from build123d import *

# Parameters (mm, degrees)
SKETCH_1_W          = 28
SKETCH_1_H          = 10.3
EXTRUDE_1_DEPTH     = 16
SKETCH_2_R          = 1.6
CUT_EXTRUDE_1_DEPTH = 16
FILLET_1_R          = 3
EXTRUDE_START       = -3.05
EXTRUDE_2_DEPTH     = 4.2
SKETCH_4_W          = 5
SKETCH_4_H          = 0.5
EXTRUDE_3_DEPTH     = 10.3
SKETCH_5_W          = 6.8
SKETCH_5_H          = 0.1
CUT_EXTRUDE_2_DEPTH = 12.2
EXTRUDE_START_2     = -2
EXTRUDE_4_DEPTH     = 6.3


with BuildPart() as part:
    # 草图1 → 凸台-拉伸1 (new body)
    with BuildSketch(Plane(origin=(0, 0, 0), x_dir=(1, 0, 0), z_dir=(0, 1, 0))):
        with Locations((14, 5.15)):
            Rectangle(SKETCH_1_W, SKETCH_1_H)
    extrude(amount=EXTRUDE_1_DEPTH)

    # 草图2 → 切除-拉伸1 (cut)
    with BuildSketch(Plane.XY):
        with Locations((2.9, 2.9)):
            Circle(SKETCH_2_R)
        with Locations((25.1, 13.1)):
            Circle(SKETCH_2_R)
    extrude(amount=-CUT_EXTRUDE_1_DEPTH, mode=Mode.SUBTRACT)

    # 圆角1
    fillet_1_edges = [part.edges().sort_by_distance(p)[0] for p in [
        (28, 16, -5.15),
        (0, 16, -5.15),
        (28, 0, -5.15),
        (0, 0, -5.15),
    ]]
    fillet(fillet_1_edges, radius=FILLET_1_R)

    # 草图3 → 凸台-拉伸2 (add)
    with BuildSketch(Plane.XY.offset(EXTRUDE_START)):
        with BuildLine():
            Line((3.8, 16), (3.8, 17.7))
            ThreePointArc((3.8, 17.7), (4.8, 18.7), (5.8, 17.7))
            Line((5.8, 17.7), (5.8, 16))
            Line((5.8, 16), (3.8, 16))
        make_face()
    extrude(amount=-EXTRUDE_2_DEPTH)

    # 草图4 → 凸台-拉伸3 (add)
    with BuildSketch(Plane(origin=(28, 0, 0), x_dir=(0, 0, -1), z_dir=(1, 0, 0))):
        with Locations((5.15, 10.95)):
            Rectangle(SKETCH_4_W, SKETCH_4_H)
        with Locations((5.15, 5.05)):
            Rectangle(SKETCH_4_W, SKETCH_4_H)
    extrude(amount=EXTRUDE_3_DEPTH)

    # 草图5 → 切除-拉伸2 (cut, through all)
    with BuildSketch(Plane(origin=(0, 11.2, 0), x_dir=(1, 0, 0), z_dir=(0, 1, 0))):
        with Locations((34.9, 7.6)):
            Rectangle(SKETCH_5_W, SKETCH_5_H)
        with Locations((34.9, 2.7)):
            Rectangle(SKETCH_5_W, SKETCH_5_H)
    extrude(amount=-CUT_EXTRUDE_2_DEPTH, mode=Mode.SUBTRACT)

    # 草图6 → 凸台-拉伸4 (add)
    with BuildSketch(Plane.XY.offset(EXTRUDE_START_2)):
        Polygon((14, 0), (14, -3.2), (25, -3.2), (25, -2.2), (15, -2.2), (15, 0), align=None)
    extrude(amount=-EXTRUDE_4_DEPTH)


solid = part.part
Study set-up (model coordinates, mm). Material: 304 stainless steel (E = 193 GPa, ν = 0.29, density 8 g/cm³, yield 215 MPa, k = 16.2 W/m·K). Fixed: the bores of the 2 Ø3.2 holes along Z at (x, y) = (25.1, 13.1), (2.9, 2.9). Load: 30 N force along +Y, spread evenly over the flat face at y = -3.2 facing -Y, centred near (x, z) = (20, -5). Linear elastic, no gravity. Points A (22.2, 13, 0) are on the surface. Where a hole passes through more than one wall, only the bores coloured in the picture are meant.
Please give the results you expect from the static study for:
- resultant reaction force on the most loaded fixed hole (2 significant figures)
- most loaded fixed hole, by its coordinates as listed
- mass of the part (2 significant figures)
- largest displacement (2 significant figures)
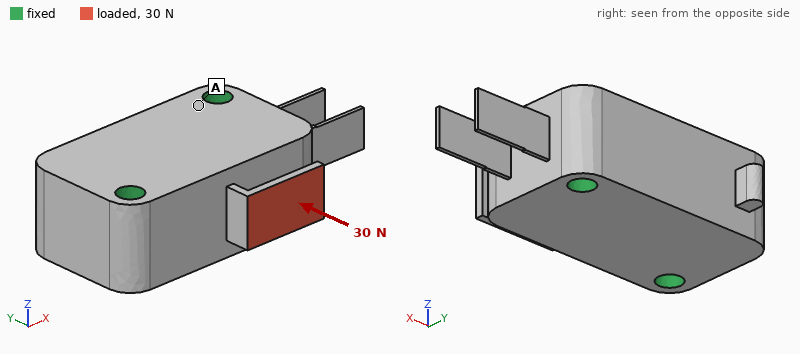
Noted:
23 N
(25.1, 13.1)
36 g
74 µm
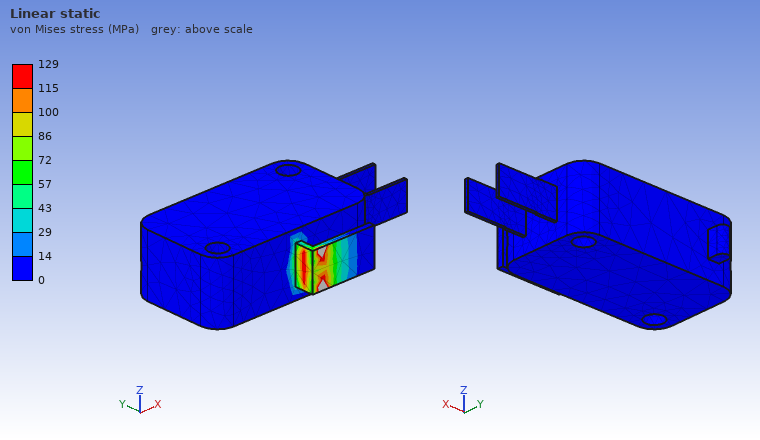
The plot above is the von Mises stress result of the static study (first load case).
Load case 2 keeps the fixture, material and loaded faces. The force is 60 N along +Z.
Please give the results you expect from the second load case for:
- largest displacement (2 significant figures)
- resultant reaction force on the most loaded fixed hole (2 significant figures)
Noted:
25 µm
31 N
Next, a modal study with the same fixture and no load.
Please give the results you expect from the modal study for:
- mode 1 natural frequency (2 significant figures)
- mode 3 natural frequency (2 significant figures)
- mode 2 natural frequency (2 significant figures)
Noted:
3800 Hz
5300 Hz
3800 Hz
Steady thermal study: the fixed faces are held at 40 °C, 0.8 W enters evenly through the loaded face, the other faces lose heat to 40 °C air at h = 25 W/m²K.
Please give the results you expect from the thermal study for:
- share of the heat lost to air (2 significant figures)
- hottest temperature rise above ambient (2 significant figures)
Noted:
20 %
55 K
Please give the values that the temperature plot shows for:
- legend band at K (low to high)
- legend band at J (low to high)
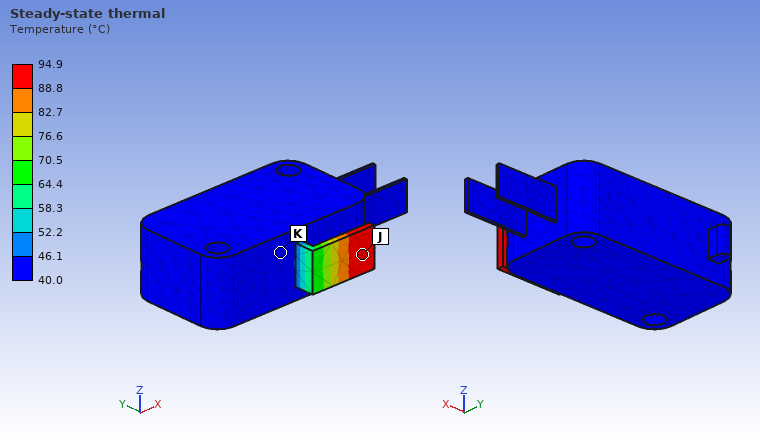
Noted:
40.0 to 46.1 °C
88.8 to 94.9 °C
